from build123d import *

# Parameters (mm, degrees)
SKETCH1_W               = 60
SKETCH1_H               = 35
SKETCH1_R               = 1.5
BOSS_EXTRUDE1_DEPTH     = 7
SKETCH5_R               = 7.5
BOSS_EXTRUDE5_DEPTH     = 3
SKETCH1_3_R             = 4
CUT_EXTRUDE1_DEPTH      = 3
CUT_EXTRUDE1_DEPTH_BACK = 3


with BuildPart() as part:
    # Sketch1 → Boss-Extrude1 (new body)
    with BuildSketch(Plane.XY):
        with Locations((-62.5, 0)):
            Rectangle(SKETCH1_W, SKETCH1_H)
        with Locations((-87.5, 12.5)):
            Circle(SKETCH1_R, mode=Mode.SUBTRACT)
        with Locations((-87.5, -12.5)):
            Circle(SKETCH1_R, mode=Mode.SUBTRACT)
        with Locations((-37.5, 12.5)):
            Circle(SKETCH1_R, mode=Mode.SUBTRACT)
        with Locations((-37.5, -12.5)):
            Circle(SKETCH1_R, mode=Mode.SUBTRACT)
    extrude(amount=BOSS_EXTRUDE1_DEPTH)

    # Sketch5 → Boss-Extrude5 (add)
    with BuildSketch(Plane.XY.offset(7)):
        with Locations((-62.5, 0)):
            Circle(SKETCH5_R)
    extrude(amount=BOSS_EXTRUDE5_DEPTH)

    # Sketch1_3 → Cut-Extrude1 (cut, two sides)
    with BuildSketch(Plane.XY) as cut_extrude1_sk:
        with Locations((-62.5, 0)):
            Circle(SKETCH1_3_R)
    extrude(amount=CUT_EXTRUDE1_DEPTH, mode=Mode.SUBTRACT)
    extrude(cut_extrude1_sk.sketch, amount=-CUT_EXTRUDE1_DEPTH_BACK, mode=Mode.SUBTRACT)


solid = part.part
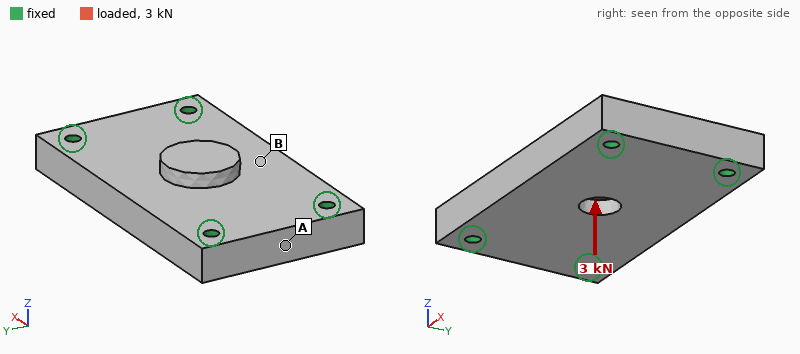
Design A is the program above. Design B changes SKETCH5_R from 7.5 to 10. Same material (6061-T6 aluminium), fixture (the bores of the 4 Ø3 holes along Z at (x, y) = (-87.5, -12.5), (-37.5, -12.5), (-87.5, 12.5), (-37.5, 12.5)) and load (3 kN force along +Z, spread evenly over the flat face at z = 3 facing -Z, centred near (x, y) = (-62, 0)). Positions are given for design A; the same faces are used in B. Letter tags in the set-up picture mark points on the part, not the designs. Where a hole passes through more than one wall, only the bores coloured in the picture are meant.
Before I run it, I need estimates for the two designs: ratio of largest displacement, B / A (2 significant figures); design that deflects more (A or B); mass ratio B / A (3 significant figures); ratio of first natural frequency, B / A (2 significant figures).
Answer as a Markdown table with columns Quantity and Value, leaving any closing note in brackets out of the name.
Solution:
| Quantity | Value |
|---|---|
| ratio of largest displacement, B / A | 0.90 |
| design that deflects more | A |
| mass ratio B / A | 1.03 |
| ratio of first natural frequency, B / A | 1.0 |
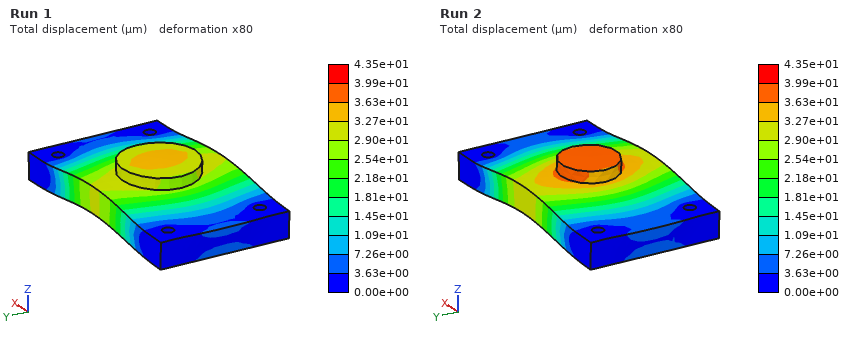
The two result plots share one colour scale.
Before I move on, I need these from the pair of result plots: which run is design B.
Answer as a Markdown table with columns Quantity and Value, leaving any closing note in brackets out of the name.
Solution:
| Quantity | Value |
|---|---|
| which run is design B | Run 1 |
